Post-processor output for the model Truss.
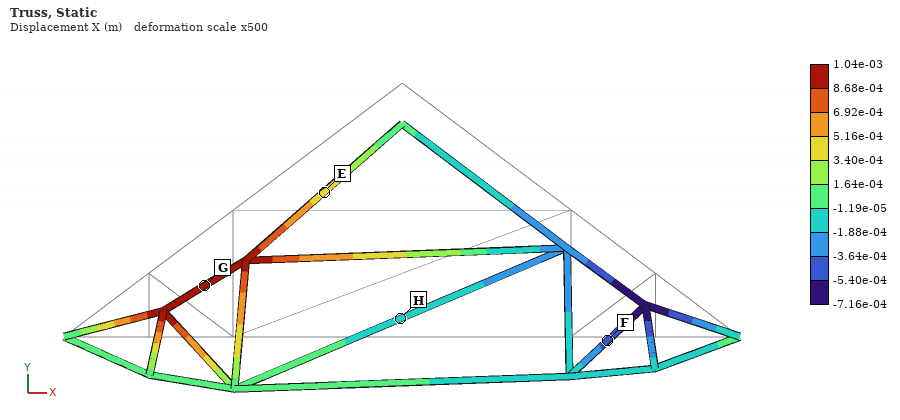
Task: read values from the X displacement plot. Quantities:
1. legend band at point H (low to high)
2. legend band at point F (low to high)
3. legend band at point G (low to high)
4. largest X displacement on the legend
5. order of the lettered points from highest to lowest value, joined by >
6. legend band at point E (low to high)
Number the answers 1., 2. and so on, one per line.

1. -1.88e-04 to -1.19e-05 m
2. -5.40e-04 to -3.64e-04 m
3. 8.68e-04 to 1.04e-03 m
4. 1.04e-03 m
5. G > E > H > F
6. 3.40e-04 to 5.16e-04 m
